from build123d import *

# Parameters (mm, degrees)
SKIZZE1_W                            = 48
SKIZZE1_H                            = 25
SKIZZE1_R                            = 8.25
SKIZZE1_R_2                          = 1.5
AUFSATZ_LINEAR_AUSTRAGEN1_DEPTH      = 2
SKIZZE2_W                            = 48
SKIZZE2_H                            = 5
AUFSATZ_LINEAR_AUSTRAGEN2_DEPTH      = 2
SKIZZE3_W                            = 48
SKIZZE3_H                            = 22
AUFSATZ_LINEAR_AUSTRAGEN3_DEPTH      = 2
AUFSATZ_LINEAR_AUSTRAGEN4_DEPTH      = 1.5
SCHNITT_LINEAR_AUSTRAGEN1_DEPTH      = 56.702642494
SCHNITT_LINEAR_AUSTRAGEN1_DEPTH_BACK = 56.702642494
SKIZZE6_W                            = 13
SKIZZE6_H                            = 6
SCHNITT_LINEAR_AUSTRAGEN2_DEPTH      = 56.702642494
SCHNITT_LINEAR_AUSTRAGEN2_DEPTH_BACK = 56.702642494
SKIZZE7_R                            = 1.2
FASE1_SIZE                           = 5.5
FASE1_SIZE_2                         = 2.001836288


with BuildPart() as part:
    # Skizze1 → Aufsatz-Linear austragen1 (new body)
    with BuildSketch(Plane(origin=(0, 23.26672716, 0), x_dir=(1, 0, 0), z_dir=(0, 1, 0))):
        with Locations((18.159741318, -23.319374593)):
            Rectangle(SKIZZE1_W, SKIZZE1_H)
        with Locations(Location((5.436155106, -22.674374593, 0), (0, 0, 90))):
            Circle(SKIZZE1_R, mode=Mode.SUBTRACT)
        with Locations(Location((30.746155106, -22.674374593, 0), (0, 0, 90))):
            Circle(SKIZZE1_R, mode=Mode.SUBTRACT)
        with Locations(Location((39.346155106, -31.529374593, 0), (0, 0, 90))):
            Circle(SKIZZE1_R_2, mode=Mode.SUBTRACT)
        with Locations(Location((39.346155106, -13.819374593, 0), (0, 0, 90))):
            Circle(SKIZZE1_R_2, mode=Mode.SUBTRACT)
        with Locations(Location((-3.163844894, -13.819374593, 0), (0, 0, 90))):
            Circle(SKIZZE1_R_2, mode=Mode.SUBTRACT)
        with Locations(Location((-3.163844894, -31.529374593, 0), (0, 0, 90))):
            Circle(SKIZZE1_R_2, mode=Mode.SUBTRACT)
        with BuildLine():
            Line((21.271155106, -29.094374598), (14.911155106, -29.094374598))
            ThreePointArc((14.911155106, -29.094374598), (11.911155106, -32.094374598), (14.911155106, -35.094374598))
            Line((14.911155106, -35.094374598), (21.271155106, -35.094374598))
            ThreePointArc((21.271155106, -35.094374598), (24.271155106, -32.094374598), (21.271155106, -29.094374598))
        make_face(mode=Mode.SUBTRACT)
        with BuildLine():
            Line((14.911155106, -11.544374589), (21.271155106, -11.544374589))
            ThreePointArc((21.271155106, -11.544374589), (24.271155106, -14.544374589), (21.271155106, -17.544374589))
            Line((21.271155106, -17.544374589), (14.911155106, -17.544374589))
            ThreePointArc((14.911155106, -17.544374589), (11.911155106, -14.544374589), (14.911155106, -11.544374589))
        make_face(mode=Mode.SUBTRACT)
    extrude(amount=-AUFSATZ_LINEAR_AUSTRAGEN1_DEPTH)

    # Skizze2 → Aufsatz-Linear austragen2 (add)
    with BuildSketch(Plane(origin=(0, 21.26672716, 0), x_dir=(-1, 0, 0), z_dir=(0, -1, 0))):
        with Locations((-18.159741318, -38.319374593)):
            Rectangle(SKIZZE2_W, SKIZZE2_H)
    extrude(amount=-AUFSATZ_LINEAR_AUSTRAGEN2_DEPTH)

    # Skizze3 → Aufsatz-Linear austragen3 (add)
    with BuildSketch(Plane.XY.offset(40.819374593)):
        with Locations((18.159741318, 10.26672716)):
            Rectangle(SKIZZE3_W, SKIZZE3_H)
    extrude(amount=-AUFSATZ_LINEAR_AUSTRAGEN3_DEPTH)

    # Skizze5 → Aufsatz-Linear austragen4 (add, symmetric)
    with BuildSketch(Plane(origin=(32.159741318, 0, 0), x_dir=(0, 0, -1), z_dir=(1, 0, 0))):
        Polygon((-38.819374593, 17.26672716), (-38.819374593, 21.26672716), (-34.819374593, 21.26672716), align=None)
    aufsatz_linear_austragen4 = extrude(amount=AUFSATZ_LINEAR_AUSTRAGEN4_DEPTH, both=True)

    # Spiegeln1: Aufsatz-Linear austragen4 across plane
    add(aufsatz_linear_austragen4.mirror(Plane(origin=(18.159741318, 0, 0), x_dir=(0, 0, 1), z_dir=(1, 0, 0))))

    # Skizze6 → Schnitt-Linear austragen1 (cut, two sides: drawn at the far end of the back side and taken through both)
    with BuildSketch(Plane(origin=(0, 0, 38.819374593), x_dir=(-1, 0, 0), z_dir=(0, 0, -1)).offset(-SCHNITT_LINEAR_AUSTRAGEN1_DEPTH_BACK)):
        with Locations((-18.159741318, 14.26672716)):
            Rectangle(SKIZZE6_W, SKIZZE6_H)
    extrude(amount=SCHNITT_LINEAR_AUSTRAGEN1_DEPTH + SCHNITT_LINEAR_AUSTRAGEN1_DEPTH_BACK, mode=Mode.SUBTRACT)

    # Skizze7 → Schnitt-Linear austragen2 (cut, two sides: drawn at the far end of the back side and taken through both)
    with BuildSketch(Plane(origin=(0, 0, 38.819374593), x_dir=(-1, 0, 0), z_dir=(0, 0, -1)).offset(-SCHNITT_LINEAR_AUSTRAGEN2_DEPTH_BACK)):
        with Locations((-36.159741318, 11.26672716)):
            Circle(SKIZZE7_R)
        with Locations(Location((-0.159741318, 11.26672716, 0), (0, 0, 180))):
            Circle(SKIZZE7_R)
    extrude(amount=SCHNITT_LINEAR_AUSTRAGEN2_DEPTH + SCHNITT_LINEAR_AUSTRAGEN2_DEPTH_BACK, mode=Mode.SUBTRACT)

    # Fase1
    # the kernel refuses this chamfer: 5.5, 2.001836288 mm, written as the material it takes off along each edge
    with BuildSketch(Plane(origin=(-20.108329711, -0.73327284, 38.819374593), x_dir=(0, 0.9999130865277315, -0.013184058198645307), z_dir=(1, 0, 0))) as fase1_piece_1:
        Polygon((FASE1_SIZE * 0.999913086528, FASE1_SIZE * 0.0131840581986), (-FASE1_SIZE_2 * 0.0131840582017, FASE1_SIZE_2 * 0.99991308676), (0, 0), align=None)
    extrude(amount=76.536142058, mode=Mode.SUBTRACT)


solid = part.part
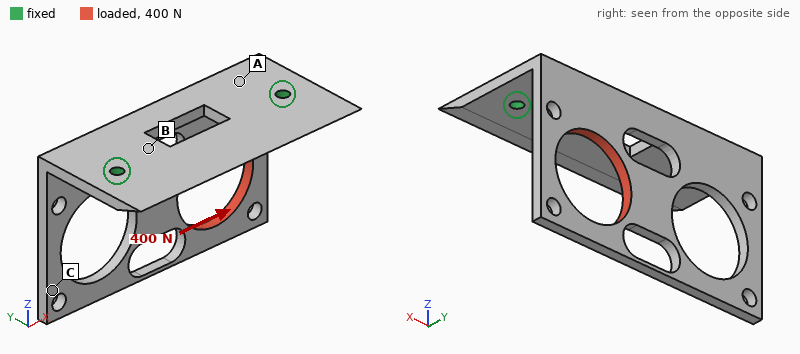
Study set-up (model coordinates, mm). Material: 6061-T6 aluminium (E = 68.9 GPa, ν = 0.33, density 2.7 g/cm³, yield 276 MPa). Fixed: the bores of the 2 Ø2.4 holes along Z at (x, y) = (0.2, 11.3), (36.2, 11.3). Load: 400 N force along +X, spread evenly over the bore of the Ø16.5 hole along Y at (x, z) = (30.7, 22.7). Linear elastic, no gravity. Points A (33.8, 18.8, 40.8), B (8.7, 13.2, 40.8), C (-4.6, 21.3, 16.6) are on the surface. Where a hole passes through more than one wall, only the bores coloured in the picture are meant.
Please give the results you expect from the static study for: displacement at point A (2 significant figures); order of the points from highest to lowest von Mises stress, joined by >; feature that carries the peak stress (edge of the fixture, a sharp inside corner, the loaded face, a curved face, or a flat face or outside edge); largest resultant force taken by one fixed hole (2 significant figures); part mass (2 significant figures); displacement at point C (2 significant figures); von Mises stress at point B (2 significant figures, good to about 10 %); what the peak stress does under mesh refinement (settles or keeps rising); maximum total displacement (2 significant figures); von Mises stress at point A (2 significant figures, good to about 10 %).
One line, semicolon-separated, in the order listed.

0.038 mm; A > B > C; edge of the fixture; 290 N; 9.2 g; 0.20 mm; 27 MPa; keeps rising; 0.23 mm; 43 MPa
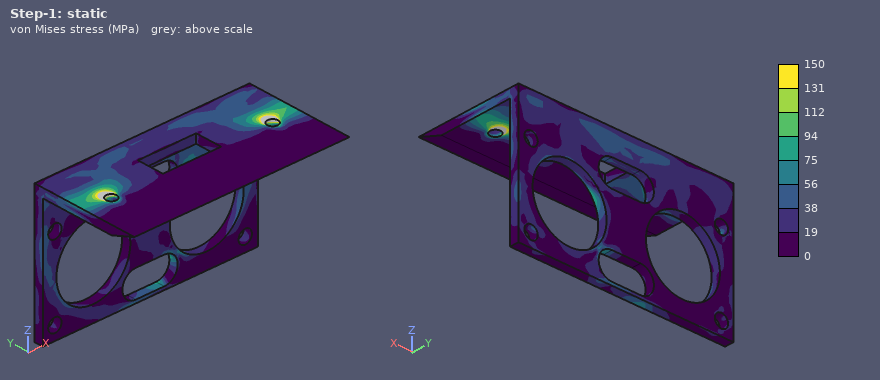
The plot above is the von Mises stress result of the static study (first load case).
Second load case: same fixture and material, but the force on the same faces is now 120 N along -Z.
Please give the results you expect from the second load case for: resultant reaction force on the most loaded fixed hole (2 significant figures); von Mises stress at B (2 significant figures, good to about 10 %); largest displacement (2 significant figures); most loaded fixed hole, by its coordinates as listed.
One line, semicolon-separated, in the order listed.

100 N; 17 MPa; 0.19 mm; (36.2, 11.3)
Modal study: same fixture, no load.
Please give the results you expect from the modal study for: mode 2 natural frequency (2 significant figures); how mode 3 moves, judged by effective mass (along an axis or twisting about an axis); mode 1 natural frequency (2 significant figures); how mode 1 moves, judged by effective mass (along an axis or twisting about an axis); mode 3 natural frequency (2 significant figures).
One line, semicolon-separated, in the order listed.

2500 Hz; along Z; 1400 Hz; along Y; 4400 Hz
